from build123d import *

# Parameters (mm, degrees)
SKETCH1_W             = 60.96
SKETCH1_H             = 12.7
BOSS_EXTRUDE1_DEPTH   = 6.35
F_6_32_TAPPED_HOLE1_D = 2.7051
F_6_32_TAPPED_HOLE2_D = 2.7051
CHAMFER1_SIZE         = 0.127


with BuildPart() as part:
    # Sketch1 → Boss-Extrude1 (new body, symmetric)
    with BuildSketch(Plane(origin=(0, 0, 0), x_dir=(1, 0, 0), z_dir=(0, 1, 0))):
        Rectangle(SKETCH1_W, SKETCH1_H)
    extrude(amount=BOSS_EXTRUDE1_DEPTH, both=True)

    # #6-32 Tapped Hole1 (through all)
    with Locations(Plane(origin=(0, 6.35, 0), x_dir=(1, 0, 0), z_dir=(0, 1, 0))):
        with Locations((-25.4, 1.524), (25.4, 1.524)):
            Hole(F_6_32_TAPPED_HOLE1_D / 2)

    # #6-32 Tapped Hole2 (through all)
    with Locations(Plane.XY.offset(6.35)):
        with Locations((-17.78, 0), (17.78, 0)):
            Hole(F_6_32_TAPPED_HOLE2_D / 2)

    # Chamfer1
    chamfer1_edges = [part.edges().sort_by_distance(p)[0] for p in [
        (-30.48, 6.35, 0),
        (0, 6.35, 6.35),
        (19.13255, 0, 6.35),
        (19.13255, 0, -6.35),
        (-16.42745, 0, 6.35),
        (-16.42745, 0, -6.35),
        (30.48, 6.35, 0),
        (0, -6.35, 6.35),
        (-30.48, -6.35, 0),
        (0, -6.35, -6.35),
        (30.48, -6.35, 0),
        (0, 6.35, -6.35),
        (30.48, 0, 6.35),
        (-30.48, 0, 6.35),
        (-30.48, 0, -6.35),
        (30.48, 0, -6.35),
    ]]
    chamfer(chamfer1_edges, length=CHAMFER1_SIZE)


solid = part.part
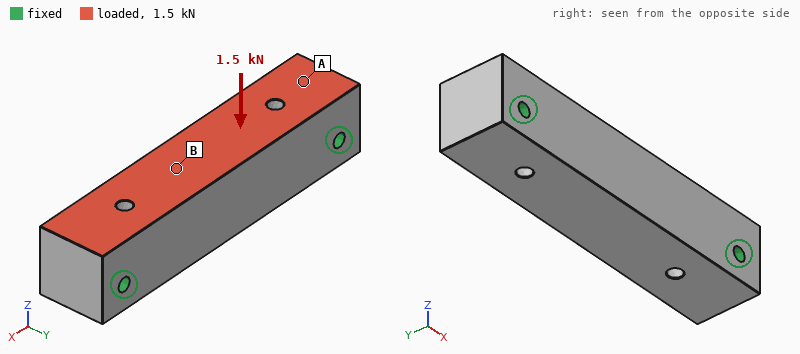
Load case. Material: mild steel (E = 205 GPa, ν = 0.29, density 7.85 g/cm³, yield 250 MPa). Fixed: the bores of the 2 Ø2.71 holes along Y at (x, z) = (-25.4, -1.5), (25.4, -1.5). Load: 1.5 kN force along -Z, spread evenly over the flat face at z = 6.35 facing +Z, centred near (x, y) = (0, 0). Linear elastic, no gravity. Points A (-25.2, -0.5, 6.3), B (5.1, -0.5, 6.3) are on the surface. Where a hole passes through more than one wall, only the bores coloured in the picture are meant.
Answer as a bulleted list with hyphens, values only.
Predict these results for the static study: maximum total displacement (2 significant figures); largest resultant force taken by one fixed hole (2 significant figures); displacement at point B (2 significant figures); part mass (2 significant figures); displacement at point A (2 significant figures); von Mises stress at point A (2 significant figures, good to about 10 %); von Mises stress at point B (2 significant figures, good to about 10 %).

- 3.0 µm
- 790 N
- 2.8 µm
- 75 g
- 0.88 µm
- 5.1 MPa
- 13 MPa
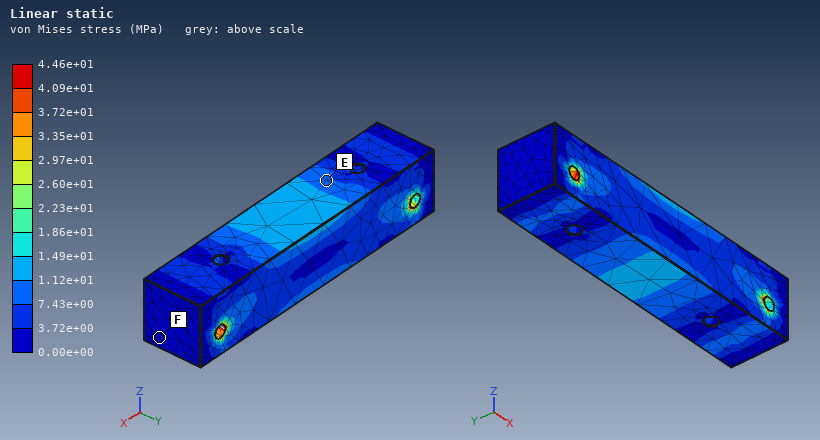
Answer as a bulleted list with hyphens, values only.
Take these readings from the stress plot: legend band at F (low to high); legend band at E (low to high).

- 0.00e+00 to 3.72e+00 MPa
- 7.43e+00 to 1.12e+01 MPa
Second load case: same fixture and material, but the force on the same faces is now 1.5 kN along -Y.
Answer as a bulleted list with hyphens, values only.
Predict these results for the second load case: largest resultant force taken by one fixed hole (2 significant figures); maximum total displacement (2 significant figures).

- 750 N
- 4.0 µm
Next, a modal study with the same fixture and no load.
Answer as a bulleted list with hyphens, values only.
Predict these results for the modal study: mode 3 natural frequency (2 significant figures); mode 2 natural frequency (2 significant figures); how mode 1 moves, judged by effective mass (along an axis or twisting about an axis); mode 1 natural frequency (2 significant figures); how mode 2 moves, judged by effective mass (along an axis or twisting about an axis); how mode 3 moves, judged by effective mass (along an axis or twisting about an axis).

- 27 kHz
- 17 kHz
- along Z
- 14 kHz
- along Y
- twisting about X
